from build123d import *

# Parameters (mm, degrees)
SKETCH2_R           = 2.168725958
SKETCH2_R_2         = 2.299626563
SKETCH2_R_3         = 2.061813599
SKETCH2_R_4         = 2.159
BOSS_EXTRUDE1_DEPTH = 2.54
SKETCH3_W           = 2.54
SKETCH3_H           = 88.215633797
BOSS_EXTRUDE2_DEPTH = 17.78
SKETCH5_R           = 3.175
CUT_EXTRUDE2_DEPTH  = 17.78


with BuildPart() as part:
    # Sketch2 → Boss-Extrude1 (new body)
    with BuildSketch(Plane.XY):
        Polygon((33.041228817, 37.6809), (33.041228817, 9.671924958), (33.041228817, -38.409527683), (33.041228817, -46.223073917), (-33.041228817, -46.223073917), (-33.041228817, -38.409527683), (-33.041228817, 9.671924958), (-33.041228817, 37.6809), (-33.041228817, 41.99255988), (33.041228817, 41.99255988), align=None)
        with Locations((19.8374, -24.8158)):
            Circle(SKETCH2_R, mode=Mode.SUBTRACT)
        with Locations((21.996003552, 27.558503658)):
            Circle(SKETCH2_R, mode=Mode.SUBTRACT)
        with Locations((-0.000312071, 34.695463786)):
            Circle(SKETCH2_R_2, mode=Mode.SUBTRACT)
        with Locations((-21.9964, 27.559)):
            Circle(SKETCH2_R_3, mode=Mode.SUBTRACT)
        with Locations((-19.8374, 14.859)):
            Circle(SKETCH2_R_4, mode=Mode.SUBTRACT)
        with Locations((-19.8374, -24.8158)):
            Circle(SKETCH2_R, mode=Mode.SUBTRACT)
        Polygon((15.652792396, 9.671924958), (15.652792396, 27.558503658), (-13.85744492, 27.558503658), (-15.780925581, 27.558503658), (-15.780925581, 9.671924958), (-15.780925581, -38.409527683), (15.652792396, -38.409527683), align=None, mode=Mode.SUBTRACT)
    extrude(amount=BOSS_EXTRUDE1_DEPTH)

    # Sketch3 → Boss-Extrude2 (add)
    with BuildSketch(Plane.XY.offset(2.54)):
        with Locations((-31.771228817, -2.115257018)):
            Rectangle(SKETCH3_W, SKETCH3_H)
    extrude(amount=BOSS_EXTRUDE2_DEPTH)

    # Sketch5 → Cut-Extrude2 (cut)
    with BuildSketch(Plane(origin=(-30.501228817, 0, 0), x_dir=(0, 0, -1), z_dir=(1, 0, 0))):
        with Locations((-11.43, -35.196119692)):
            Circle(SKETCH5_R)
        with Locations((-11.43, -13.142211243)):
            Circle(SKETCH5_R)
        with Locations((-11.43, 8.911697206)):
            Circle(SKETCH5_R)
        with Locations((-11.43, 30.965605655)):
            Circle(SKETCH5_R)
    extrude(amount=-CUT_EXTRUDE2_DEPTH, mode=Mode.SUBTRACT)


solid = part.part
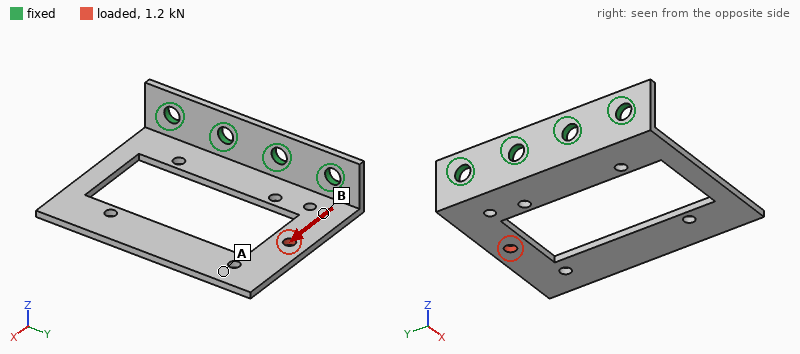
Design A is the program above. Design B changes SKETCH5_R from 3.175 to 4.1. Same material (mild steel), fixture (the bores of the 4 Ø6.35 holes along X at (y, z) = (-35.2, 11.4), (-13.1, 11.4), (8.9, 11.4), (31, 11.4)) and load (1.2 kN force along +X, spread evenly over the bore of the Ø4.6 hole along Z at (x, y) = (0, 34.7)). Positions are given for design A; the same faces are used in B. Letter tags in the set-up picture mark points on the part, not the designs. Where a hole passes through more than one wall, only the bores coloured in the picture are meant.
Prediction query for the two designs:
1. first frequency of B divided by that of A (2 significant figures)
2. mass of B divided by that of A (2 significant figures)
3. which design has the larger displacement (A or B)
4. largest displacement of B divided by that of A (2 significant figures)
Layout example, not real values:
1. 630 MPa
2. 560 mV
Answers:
1. 1.0
2. 0.98
3. A
4. 0.79
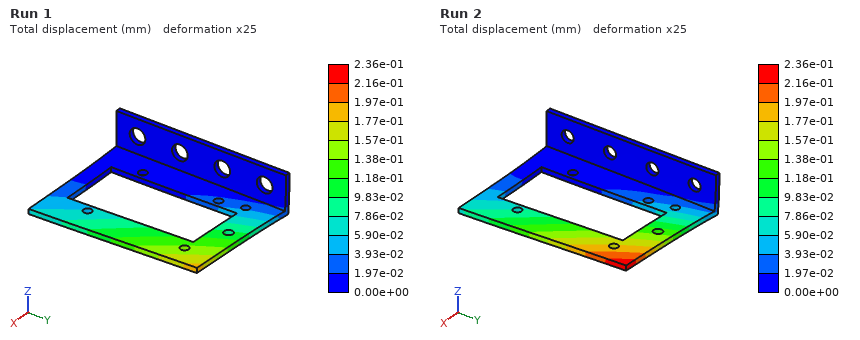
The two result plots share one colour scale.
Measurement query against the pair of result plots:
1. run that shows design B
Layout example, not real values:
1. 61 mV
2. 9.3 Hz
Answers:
1. Run 1
